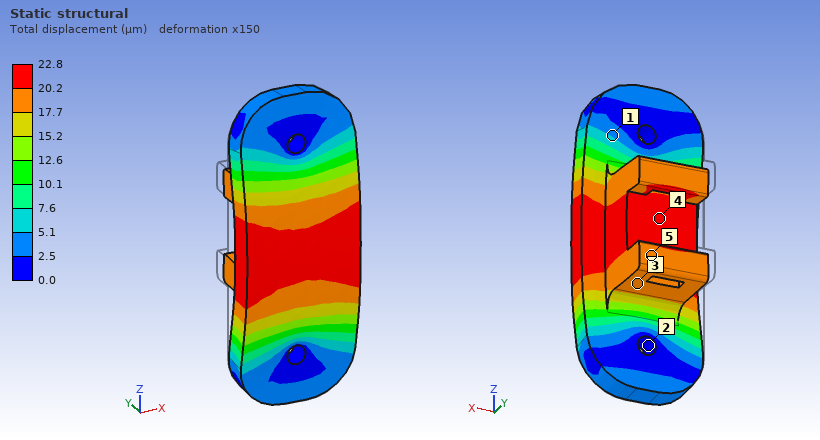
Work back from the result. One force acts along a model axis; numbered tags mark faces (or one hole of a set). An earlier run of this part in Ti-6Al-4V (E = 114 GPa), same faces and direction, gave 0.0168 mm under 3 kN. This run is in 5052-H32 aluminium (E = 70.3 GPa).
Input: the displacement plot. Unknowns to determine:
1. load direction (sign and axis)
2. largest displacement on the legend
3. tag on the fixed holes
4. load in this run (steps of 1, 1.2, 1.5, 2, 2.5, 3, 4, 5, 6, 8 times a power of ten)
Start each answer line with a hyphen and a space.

- -Y
- 22.8 µm
- 2
- 2.5 kN
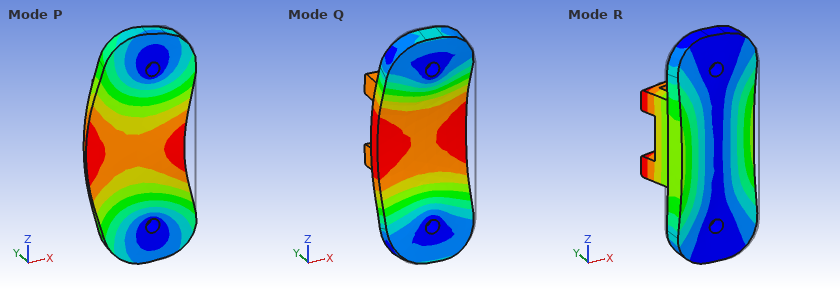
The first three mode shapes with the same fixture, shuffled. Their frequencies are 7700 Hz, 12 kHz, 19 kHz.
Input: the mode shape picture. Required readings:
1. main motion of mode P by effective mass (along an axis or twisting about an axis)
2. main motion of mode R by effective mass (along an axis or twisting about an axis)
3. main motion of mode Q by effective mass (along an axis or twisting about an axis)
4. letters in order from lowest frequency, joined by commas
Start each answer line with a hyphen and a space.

- along X
- along X
- along Y
- R, Q, P
